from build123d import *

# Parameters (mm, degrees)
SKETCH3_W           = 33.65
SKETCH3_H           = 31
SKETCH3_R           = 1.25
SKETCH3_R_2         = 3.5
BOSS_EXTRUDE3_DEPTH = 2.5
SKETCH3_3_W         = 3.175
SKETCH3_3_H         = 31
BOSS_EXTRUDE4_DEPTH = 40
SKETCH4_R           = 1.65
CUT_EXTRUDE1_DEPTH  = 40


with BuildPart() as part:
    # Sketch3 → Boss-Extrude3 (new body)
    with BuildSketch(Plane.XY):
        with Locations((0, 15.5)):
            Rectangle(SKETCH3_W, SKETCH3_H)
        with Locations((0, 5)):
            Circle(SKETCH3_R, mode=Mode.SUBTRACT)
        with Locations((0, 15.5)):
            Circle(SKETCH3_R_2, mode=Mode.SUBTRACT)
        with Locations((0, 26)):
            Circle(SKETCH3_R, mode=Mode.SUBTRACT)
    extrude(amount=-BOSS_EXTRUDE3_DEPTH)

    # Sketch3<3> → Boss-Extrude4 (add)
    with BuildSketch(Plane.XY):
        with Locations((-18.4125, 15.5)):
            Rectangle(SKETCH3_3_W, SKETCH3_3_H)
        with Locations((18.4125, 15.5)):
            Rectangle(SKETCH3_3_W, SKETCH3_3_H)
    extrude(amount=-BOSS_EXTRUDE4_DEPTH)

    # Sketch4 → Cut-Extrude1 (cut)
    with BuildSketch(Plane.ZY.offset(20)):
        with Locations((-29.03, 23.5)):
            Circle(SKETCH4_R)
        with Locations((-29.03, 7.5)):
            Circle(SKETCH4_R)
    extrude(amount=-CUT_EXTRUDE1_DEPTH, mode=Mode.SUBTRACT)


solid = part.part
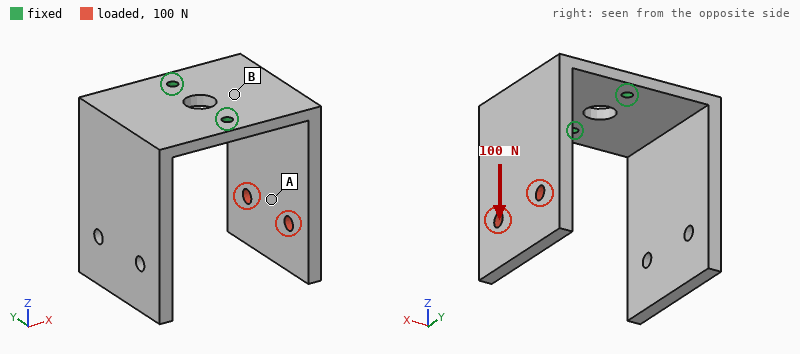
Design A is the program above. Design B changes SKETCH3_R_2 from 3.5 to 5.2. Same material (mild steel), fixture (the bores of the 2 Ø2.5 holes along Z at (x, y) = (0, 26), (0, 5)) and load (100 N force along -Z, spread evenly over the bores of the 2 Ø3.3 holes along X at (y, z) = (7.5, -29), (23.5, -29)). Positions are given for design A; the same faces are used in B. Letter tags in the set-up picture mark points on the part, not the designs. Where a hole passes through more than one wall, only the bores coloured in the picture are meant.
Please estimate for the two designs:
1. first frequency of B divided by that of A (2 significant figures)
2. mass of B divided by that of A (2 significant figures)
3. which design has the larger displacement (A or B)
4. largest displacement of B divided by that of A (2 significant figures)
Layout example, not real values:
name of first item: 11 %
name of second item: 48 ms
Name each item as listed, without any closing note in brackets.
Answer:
first frequency of B divided by that of A: 0.98
mass of B divided by that of A: 0.99
which design has the larger displacement: B
largest displacement of B divided by that of A: 1.1
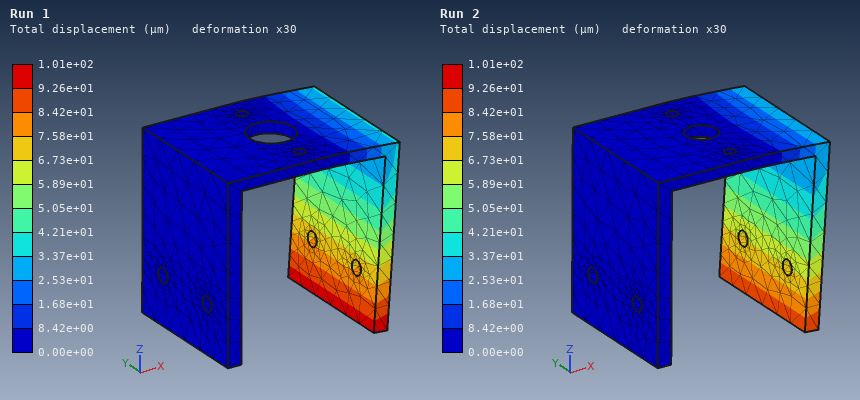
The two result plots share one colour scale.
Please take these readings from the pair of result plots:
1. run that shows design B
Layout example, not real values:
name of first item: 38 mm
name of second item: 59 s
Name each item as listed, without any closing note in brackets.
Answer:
run that shows design B: Run 1
